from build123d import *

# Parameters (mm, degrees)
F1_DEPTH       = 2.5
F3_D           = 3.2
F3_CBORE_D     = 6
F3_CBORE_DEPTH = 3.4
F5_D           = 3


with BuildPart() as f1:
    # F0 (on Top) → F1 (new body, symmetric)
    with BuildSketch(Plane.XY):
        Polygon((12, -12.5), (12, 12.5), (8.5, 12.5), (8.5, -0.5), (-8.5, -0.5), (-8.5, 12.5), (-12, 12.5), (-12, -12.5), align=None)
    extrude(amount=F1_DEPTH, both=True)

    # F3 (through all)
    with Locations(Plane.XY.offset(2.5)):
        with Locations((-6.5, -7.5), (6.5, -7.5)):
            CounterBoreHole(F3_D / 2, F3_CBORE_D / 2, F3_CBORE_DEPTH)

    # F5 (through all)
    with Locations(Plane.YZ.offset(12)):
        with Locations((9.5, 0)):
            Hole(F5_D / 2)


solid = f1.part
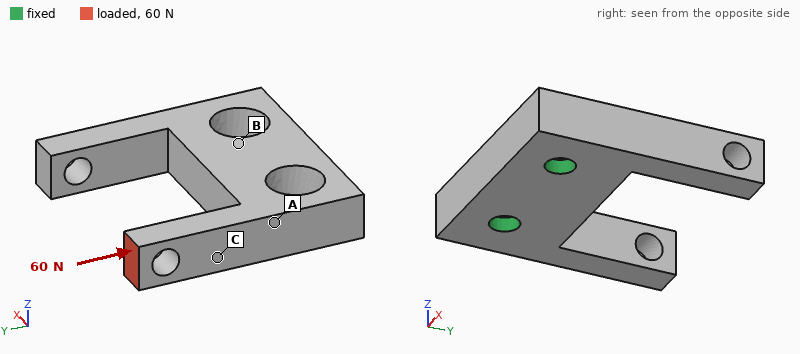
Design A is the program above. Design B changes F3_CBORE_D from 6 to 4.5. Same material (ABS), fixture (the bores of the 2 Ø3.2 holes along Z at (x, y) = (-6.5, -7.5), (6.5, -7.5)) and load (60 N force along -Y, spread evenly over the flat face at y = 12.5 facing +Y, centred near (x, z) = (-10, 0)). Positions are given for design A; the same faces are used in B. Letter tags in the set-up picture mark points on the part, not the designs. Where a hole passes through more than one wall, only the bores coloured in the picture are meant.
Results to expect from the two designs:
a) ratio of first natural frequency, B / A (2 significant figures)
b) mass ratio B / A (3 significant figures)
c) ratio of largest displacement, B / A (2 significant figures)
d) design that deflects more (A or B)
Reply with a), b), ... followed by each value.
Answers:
a) 1.1
b) 1.05
c) 0.84
d) A
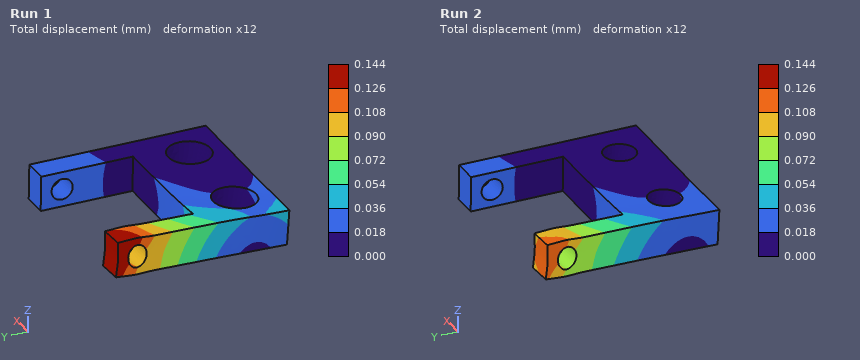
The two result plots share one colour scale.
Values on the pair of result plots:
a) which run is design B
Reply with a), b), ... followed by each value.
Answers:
a) Run 2
